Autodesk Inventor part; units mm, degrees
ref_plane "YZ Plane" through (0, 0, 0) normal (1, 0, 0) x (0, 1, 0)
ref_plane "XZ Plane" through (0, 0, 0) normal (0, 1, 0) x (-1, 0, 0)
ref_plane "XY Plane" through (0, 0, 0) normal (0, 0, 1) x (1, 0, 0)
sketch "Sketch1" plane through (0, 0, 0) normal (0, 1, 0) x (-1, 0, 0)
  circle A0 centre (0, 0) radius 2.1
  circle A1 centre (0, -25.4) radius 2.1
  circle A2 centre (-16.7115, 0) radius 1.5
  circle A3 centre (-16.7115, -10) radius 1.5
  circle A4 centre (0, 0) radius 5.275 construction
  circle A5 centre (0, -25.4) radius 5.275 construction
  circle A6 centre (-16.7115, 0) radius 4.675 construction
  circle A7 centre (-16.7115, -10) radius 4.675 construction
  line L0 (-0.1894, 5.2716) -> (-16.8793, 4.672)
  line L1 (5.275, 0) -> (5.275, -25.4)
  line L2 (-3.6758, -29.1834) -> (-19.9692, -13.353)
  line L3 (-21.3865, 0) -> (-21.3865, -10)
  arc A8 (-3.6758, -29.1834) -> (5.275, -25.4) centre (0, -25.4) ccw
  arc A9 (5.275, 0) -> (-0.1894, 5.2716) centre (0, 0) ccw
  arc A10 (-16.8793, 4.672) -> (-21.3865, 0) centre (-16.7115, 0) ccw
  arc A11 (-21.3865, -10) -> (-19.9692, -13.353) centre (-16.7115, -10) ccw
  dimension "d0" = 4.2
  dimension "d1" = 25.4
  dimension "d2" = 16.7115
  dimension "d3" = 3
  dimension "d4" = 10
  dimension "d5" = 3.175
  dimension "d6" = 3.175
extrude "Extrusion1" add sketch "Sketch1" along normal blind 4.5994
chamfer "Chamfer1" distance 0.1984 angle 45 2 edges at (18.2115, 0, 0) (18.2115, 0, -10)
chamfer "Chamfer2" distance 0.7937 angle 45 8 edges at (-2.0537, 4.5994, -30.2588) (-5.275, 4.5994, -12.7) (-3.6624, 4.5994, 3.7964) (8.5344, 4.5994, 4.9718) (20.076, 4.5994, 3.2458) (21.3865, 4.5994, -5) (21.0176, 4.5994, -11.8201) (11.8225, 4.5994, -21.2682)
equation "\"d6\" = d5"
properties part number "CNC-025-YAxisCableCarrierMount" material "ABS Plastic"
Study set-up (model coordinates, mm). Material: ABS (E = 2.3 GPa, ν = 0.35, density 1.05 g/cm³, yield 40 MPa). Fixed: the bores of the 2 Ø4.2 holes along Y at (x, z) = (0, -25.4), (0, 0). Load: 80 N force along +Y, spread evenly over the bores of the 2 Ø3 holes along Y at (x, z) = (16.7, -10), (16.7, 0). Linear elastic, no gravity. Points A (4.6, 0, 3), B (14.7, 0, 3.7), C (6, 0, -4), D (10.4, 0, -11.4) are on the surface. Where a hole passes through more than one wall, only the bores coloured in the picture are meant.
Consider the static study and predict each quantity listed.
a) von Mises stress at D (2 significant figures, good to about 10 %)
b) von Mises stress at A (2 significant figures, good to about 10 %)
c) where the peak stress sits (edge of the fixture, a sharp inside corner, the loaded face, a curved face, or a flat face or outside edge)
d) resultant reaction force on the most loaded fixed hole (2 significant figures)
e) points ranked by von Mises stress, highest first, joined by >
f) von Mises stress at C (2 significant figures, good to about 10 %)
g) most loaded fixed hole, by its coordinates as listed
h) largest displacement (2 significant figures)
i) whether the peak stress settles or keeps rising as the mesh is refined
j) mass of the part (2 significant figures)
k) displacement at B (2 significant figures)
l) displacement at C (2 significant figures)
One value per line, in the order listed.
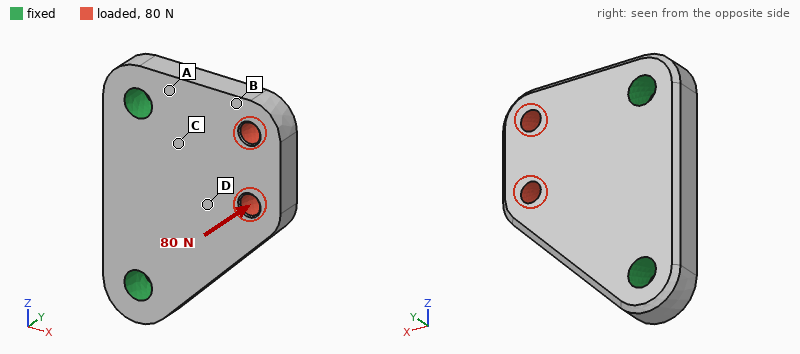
6.1 MPa
12 MPa
edge of the fixture
66 N
A > C > D > B
8.7 MPa
(0, 0)
0.42 mm
keeps rising
3.4 g
0.24 mm
0.071 mm
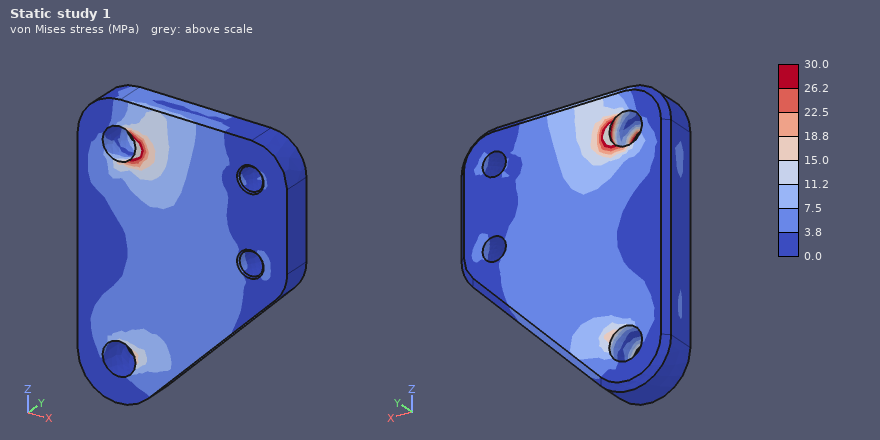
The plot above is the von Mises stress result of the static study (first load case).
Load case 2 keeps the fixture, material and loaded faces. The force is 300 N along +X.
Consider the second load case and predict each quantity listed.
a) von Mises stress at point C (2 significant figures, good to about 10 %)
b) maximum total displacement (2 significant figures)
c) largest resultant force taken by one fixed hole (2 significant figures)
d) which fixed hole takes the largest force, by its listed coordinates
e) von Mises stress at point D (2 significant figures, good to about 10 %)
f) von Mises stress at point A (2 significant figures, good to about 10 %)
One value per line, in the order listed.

3.6 MPa
41 µm
240 N
(0, 0)
1.8 MPa
3.4 MPa
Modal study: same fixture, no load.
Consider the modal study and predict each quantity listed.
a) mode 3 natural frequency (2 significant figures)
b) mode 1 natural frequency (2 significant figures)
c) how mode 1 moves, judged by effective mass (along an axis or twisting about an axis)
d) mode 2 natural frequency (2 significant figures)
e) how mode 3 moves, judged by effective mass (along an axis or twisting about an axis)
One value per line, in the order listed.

10000 Hz
2700 Hz
along Y
6200 Hz
along Z
